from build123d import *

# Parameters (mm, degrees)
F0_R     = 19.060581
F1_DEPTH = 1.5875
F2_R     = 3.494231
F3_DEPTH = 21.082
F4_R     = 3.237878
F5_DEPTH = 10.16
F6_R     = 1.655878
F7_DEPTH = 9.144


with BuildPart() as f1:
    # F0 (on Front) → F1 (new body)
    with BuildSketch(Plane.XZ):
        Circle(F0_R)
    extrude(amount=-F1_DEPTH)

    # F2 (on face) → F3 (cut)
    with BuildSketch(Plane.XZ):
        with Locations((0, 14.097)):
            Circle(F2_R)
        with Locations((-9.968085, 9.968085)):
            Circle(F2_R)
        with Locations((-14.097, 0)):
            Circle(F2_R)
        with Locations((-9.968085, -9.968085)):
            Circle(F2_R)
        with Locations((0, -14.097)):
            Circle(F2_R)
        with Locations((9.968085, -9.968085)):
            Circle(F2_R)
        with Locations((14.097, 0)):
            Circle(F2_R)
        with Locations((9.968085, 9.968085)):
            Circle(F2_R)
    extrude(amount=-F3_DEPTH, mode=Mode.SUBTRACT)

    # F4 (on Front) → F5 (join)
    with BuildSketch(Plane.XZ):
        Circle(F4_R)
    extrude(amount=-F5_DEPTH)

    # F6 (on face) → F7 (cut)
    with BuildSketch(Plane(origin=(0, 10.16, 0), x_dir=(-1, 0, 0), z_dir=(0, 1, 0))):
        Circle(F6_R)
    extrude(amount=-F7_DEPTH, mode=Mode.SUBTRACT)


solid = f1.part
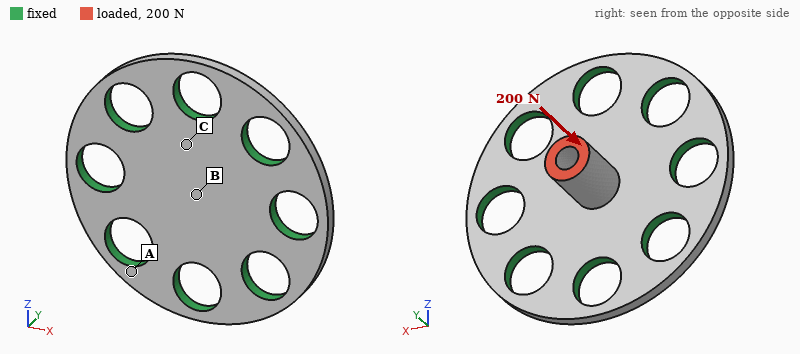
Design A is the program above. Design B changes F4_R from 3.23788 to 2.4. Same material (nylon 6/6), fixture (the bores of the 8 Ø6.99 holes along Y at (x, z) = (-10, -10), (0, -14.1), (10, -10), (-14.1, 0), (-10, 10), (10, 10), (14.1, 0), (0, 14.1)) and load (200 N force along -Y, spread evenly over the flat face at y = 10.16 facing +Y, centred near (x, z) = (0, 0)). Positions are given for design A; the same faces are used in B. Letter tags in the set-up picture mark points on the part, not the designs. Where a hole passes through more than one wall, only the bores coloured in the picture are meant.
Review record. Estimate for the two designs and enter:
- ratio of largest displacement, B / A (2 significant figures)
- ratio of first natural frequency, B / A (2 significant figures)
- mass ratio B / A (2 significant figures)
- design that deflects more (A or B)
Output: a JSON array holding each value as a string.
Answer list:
["1.5", "1.1", "0.92", "B"]
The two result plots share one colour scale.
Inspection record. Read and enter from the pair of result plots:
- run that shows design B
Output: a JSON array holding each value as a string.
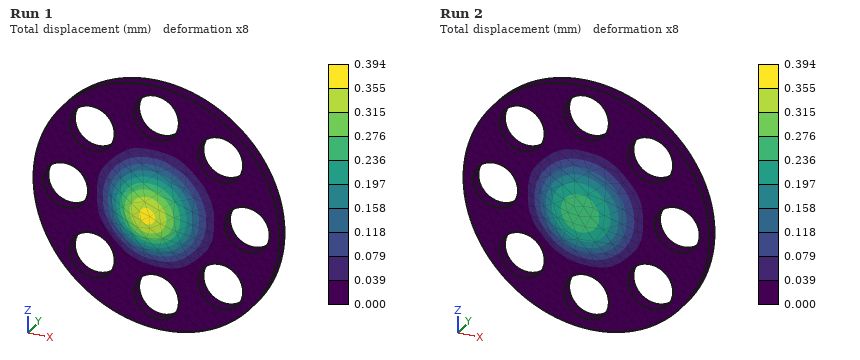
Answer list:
["Run 1"]
